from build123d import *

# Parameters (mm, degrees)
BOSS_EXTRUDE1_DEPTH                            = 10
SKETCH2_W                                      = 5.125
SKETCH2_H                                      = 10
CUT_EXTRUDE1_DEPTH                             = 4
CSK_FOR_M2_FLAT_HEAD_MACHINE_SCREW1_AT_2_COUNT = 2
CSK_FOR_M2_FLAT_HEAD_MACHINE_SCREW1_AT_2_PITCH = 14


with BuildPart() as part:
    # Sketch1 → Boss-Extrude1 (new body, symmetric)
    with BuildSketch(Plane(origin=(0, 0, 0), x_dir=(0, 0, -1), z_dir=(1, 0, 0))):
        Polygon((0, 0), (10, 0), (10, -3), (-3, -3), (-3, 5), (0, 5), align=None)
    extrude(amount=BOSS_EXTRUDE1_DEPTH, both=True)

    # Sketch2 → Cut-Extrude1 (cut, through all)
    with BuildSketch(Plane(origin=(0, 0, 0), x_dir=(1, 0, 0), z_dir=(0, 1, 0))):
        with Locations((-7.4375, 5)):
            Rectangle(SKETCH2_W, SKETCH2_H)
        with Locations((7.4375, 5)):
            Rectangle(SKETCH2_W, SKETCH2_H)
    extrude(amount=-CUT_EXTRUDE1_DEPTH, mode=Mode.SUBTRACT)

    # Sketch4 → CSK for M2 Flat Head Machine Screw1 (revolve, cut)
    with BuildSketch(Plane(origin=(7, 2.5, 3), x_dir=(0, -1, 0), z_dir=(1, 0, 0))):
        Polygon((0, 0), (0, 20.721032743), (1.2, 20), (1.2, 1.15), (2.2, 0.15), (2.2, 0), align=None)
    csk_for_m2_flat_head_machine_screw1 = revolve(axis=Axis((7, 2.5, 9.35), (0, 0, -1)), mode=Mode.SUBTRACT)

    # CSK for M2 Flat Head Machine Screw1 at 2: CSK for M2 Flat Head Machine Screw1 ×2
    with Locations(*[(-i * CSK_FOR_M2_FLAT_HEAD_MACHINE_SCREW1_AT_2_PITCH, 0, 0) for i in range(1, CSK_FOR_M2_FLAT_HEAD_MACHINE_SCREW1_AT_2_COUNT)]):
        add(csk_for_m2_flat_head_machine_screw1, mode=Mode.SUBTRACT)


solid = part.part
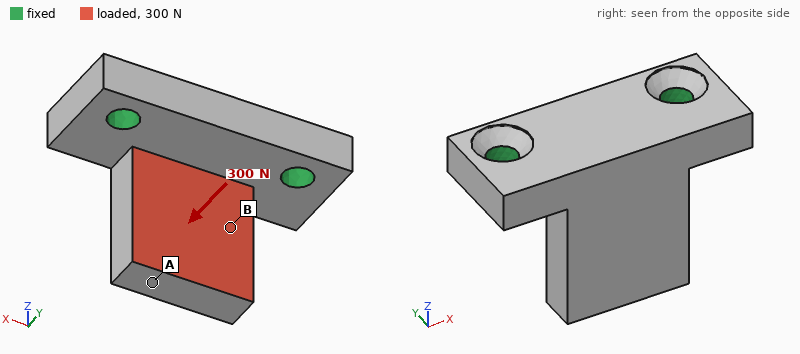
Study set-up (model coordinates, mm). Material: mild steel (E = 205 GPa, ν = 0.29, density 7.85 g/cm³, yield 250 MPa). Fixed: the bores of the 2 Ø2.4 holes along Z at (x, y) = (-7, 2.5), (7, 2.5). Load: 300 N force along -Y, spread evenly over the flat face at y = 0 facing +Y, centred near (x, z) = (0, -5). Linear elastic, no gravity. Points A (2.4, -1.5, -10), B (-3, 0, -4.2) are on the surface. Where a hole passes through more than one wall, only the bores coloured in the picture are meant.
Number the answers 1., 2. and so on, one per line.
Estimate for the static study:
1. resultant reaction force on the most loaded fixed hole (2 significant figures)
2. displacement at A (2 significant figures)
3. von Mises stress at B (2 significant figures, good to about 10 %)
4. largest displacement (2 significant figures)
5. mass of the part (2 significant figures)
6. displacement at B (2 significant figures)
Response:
1. 160 N
2. 30 µm
3. 38 MPa
4. 31 µm
5. 5.8 g
6. 13 µm
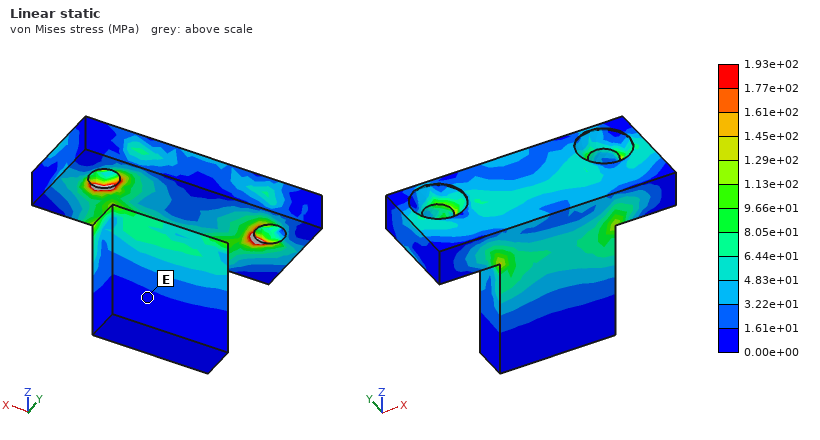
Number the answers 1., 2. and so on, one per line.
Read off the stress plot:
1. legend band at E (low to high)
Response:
1. 0.00e+00 to 1.61e+01 MPa
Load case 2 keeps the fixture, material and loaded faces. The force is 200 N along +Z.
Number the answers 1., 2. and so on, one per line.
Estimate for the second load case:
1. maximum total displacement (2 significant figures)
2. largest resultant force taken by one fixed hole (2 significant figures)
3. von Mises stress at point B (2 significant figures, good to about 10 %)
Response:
1. 1.8 µm
2. 100 N
3. 16 MPa
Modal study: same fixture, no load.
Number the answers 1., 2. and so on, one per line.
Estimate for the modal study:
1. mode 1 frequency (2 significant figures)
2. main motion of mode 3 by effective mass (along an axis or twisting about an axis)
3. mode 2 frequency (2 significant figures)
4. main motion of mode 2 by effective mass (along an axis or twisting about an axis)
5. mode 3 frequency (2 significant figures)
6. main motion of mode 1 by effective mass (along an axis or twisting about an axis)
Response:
1. 12 kHz
2. along Z
3. 27 kHz
4. along X
5. 34 kHz
6. along Y
